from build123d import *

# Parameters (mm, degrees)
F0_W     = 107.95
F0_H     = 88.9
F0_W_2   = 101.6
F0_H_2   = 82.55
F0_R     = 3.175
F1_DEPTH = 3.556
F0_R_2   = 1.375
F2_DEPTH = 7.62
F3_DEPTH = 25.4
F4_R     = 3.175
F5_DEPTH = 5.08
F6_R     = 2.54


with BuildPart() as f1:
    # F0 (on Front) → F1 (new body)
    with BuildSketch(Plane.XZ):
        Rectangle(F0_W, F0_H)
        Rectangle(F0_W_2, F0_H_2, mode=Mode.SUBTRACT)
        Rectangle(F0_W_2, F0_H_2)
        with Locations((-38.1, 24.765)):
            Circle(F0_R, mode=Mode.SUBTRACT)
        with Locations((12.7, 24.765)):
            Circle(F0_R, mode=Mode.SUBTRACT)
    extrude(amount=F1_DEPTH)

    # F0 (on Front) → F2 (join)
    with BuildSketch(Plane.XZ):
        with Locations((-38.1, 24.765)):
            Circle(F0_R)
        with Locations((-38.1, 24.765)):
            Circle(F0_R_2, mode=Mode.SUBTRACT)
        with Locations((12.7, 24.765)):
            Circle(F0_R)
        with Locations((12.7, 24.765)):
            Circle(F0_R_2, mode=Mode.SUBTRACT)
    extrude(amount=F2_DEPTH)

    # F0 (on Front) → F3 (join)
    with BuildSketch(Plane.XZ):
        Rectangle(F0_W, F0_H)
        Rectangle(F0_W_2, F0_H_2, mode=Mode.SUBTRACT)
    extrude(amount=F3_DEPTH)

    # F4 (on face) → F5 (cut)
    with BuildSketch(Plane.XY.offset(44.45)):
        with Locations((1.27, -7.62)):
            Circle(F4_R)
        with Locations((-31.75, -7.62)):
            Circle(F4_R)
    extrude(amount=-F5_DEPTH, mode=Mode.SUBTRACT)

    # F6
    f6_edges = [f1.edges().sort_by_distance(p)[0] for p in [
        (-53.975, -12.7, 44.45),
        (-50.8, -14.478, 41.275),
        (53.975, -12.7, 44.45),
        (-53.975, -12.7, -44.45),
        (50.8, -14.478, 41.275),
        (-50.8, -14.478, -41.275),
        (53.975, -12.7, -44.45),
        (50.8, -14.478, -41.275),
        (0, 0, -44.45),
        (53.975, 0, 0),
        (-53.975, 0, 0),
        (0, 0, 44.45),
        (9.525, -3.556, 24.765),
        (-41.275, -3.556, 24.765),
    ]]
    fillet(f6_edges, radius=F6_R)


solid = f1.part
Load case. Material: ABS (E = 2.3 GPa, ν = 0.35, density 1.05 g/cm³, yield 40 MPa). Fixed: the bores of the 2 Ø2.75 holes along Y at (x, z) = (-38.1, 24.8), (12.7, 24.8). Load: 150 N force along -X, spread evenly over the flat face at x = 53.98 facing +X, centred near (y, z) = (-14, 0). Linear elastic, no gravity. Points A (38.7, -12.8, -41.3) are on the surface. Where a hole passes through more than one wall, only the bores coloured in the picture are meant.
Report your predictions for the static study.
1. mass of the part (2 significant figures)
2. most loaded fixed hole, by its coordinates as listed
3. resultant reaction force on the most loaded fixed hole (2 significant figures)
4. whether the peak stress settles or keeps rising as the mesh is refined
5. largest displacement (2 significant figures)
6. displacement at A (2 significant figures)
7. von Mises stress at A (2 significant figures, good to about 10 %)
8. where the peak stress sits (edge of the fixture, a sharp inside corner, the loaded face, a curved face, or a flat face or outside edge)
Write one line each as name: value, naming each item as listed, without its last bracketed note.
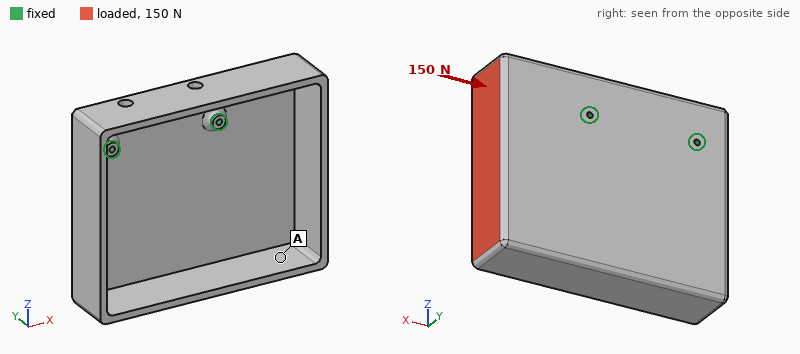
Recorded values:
mass of the part: 63 g
most loaded fixed hole, by its coordinates as listed: (12.7, 24.8)
resultant reaction force on the most loaded fixed hole: 110 N
whether the peak stress settles or keeps rising as the mesh is refined: keeps rising
largest displacement: 1.4 mm
displacement at A: 1.1 mm
von Mises stress at A: 1.1 MPa
where the peak stress sits: a sharp inside corner
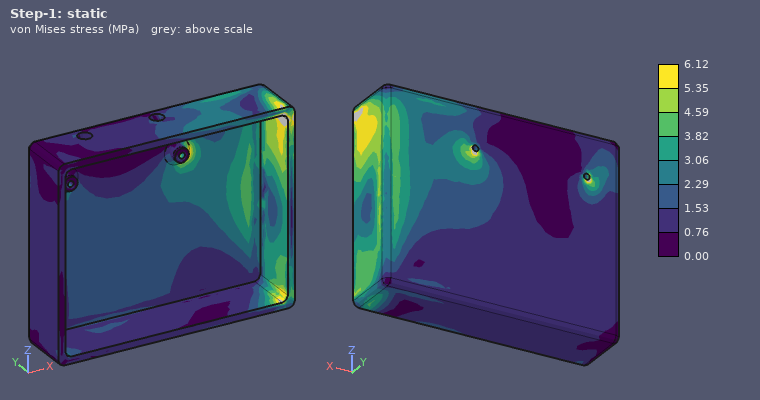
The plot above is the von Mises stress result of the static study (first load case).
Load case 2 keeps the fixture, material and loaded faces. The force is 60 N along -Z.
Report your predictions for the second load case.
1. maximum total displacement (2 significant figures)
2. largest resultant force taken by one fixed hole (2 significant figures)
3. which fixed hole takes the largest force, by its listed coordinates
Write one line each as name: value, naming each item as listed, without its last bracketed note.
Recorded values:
maximum total displacement: 1.4 mm
largest resultant force taken by one fixed hole: 110 N
which fixed hole takes the largest force, by its listed coordinates: (12.7, 24.8)
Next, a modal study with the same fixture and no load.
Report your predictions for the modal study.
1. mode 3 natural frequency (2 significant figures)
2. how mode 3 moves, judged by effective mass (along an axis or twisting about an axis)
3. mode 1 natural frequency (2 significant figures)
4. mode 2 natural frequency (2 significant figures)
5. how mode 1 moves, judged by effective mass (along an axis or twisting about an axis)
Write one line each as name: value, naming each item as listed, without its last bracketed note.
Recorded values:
mode 3 natural frequency: 560 Hz
how mode 3 moves, judged by effective mass: along Y
mode 1 natural frequency: 140 Hz
mode 2 natural frequency: 250 Hz
how mode 1 moves, judged by effective mass: along Y
